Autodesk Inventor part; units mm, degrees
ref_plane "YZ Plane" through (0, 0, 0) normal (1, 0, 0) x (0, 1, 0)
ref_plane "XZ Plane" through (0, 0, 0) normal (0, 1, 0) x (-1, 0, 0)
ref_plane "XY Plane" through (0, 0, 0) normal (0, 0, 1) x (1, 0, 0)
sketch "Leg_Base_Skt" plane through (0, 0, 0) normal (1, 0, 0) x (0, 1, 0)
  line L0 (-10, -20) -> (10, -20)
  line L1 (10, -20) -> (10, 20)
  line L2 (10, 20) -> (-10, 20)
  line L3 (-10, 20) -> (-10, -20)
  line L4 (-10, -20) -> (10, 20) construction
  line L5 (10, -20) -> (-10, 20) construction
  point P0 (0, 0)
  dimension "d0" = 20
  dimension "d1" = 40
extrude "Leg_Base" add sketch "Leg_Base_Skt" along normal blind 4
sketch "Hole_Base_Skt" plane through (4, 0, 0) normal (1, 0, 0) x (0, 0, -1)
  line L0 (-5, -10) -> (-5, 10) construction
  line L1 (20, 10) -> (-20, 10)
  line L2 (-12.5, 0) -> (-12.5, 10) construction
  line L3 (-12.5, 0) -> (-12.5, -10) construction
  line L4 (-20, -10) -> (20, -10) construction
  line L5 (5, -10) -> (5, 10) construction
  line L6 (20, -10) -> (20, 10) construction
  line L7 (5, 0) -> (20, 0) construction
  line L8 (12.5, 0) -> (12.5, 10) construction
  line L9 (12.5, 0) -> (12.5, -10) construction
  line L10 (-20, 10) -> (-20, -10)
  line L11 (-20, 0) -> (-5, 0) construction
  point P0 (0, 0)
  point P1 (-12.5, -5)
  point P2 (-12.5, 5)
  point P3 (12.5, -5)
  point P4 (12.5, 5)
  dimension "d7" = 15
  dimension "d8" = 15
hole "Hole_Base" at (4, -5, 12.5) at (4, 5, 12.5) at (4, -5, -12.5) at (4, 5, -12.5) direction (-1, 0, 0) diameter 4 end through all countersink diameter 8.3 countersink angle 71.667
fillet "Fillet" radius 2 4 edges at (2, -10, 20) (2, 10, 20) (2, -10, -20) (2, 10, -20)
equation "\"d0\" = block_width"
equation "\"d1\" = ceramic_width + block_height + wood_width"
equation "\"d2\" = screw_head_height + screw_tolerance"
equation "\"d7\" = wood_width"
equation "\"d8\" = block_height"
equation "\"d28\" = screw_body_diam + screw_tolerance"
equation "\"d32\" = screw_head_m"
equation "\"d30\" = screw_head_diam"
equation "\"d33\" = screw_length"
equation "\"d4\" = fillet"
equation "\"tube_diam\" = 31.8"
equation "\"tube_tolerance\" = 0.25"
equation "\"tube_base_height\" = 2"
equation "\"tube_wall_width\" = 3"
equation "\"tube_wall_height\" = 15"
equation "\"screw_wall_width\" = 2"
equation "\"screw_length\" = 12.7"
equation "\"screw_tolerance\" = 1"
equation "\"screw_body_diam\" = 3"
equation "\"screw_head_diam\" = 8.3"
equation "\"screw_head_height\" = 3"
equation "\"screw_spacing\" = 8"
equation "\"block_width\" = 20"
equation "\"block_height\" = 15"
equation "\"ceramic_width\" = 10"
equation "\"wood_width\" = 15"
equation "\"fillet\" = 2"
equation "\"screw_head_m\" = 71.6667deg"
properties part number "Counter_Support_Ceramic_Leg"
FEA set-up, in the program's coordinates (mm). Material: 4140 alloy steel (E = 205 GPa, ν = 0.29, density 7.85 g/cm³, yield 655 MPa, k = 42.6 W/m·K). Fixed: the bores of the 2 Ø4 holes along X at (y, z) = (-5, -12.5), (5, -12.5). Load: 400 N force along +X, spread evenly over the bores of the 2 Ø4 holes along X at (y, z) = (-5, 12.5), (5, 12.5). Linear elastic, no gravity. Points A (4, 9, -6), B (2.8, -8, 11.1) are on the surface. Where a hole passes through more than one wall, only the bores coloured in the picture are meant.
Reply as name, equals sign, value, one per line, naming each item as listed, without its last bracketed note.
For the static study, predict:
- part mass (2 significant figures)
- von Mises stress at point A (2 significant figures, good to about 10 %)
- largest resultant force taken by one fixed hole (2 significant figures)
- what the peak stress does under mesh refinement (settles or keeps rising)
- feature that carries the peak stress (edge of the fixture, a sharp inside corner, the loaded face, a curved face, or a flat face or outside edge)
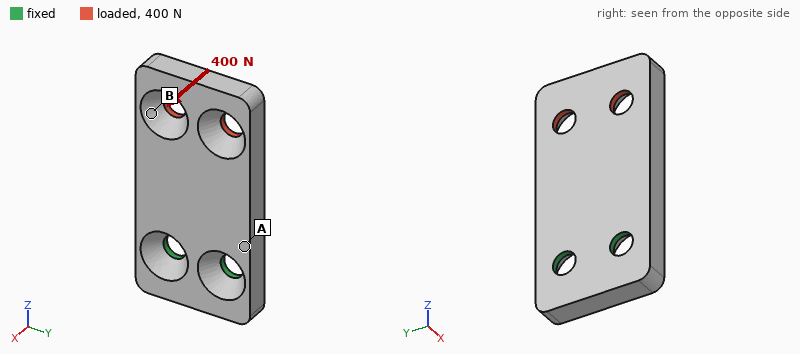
part mass = 22 g
von Mises stress at point A = 170 MPa
largest resultant force taken by one fixed hole = 250 N
what the peak stress does under mesh refinement = keeps rising
feature that carries the peak stress = edge of the fixture
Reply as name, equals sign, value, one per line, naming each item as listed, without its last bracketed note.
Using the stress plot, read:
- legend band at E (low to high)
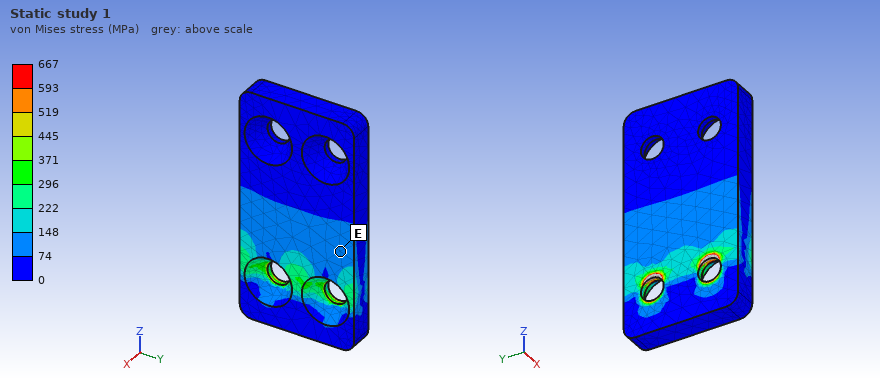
legend band at E = 74 to 148 MPa
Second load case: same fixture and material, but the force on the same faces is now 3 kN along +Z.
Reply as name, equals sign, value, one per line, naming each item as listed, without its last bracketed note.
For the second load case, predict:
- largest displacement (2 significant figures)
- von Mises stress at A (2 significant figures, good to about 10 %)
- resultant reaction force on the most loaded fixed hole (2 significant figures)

largest displacement = 97 µm
von Mises stress at A = 55 MPa
resultant reaction force on the most loaded fixed hole = 1.5 kN
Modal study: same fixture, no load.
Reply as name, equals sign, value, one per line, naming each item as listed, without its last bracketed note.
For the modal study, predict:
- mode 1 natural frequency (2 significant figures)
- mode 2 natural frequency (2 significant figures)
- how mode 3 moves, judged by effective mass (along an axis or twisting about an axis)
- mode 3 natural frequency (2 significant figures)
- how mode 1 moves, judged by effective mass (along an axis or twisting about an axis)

mode 1 natural frequency = 2500 Hz
mode 2 natural frequency = 9100 Hz
how mode 3 moves, judged by effective mass = along Y
mode 3 natural frequency = 11 kHz
how mode 1 moves, judged by effective mass = along X
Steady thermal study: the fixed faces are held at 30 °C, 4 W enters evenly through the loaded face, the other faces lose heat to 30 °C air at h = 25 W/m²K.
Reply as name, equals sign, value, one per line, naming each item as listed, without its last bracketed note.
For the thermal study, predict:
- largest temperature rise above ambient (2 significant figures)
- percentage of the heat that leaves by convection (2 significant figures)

largest temperature rise above ambient = 34 K
percentage of the heat that leaves by convection = 19 %
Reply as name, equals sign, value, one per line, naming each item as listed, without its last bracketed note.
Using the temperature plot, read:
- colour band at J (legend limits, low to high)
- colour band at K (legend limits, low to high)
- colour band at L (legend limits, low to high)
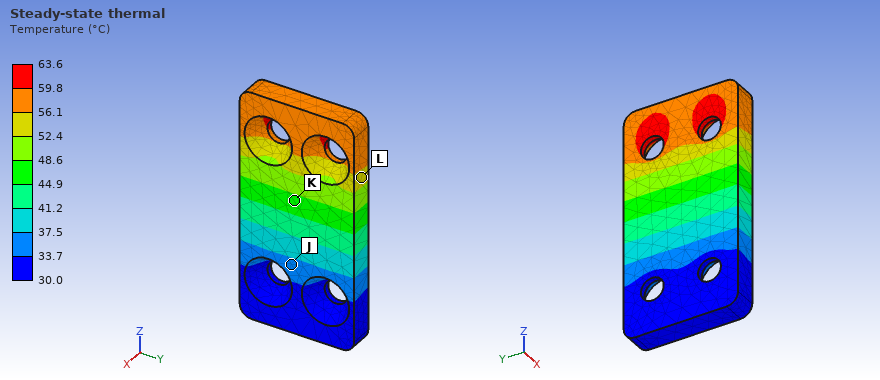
colour band at J = 33.7 to 37.5 °C
colour band at K = 44.9 to 48.6 °C
colour band at L = 52.4 to 56.1 °C
